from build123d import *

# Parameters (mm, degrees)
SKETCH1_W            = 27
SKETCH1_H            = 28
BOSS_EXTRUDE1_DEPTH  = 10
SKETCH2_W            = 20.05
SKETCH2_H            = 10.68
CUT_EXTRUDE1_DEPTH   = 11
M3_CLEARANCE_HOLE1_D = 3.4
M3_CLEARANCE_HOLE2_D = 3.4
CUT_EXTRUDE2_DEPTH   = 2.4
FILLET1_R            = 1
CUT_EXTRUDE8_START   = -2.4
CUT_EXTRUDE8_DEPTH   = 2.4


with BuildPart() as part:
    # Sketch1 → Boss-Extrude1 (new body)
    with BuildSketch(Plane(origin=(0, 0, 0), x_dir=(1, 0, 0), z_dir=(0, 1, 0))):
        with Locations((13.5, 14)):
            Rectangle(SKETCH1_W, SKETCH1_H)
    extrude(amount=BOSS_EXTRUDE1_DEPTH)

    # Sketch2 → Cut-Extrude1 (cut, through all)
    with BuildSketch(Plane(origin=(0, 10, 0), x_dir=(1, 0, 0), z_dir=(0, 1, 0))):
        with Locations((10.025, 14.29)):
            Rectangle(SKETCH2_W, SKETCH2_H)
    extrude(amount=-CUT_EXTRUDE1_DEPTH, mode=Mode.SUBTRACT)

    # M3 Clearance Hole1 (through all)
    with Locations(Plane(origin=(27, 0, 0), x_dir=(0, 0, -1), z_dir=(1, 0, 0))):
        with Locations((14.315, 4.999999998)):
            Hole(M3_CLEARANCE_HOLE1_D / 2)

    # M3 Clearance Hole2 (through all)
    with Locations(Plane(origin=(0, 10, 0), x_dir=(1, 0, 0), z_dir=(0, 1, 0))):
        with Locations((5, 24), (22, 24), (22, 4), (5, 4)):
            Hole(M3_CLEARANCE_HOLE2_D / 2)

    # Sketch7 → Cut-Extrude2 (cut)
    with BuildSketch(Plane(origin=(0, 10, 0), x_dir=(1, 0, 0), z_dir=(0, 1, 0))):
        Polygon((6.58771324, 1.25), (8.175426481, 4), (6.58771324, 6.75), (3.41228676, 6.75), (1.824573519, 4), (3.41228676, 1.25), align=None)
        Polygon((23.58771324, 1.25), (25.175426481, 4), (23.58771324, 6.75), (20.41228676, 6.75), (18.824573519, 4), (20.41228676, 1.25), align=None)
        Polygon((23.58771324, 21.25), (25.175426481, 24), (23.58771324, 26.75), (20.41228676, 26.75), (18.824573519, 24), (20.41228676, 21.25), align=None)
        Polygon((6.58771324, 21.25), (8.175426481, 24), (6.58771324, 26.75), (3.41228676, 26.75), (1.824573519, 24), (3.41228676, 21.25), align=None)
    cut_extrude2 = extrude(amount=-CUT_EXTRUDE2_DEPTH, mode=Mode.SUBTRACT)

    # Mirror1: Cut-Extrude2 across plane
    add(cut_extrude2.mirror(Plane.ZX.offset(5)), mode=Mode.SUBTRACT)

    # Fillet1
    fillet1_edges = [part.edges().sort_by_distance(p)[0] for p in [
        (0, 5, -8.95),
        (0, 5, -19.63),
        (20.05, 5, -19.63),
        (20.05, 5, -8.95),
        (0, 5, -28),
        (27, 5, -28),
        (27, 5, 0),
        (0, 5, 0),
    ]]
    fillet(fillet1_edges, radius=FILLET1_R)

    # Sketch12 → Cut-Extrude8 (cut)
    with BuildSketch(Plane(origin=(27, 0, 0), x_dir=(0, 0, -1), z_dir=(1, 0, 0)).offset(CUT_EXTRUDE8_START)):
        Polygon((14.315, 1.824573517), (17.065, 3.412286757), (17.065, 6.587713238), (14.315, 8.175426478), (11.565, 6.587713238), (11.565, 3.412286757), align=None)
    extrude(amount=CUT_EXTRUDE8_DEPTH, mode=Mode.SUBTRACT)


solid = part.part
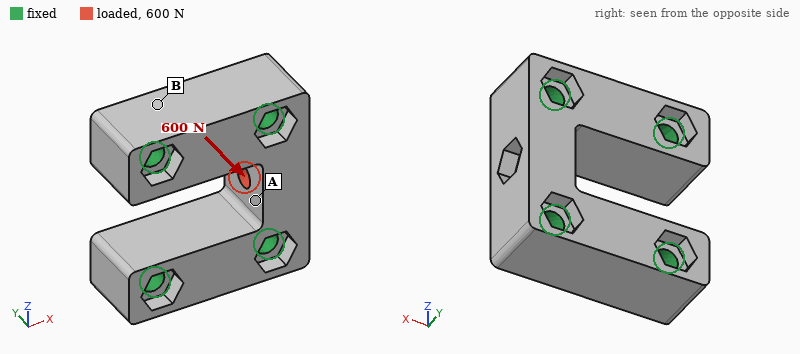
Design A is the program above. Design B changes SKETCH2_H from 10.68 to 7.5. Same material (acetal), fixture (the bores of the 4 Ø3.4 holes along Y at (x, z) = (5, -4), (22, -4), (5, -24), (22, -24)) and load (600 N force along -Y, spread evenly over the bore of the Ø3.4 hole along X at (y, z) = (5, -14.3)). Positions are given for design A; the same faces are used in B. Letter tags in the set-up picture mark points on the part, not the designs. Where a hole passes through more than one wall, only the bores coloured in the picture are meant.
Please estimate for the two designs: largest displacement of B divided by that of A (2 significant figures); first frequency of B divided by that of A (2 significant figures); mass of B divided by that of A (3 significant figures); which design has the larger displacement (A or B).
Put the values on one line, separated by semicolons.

0.91; 0.89; 1.14; A
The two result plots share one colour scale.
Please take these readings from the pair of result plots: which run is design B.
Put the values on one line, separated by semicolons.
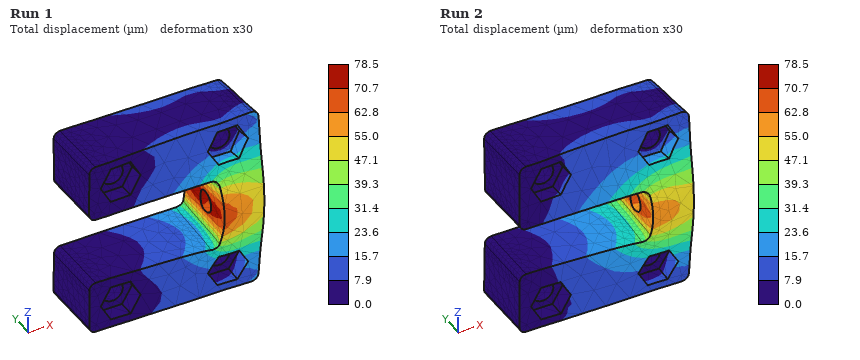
Run 2
